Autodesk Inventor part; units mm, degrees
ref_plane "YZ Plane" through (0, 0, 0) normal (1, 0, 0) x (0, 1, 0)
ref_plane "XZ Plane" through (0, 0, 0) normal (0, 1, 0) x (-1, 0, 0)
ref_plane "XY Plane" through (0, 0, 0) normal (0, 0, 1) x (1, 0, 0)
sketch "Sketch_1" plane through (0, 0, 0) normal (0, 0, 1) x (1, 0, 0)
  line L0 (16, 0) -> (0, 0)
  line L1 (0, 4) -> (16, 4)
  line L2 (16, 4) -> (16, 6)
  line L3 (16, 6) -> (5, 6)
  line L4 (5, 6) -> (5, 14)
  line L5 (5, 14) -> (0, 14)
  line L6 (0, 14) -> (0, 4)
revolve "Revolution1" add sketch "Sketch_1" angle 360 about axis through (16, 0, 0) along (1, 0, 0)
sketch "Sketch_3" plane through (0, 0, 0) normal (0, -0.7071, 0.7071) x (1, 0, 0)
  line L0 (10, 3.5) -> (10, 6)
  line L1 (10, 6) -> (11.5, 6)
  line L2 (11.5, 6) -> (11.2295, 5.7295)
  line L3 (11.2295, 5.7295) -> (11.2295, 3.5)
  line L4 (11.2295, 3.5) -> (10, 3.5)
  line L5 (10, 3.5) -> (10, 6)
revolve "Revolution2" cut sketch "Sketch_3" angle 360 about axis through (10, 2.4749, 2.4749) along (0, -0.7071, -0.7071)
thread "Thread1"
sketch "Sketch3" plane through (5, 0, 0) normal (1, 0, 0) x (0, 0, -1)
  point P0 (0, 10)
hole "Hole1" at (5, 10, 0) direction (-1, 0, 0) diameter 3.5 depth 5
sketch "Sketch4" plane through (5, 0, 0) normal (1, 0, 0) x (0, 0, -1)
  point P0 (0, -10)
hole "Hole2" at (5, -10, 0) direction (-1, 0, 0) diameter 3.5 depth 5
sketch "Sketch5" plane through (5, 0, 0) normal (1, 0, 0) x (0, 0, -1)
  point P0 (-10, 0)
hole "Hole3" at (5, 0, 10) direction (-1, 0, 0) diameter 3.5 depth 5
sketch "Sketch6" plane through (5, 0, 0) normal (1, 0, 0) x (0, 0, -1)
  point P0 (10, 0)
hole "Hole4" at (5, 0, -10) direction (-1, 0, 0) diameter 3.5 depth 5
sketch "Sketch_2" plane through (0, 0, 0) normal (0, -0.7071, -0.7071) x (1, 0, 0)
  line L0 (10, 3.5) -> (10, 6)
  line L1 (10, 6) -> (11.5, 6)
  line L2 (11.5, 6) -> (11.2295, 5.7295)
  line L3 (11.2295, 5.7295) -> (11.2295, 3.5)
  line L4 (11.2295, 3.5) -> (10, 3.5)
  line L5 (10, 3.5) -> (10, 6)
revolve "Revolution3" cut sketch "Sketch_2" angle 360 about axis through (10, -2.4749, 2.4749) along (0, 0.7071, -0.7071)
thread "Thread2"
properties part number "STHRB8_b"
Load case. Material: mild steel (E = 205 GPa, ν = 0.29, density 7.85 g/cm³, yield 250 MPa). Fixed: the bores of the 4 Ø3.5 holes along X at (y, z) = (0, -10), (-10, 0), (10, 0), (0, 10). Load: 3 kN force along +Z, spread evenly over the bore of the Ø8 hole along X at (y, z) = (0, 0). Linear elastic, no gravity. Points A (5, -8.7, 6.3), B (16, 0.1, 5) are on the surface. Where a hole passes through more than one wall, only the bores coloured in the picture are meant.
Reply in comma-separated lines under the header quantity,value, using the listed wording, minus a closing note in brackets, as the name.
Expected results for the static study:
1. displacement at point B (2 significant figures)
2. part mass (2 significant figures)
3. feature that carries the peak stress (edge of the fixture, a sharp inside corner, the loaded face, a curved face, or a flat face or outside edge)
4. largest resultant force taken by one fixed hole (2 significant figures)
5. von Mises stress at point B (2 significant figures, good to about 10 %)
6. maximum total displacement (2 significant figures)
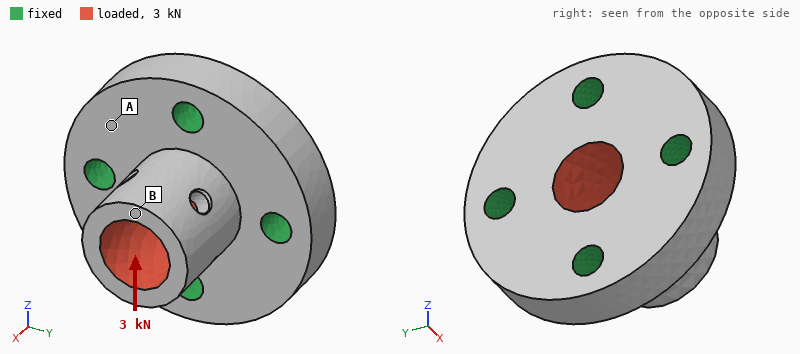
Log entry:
quantity,value
displacement at point B,11 µm
part mass,26 g
feature that carries the peak stress,the loaded face
largest resultant force taken by one fixed hole,1.3 kN
von Mises stress at point B,35 MPa
maximum total displacement,11 µm
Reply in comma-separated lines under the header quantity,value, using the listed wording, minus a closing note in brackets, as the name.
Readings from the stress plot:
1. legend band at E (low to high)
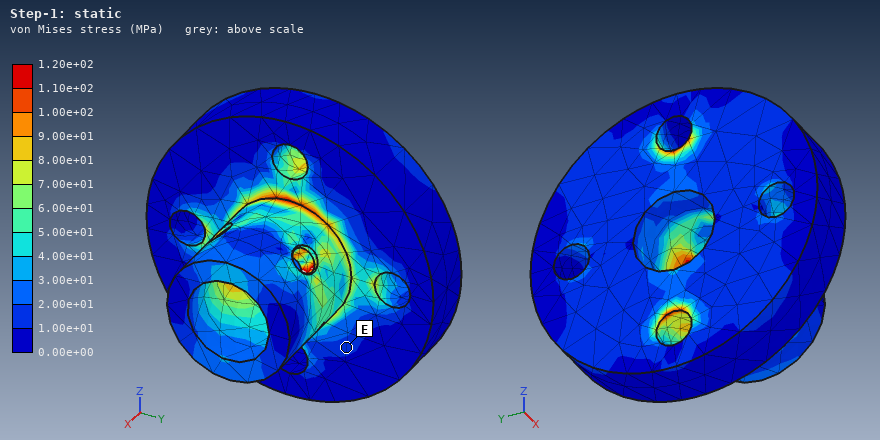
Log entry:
quantity,value
legend band at E,1.00e+01 to 2.00e+01 MPa
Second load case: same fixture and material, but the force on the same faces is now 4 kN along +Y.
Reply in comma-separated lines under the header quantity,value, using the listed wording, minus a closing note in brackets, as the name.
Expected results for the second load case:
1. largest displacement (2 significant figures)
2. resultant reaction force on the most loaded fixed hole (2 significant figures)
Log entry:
quantity,value
largest displacement,15 µm
resultant reaction force on the most loaded fixed hole,1.7 kN
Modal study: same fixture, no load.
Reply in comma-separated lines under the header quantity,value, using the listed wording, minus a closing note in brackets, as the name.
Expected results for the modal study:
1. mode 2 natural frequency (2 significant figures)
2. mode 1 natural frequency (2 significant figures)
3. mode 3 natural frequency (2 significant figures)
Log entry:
quantity,value
mode 2 natural frequency,34 kHz
mode 1 natural frequency,34 kHz
mode 3 natural frequency,55 kHz
